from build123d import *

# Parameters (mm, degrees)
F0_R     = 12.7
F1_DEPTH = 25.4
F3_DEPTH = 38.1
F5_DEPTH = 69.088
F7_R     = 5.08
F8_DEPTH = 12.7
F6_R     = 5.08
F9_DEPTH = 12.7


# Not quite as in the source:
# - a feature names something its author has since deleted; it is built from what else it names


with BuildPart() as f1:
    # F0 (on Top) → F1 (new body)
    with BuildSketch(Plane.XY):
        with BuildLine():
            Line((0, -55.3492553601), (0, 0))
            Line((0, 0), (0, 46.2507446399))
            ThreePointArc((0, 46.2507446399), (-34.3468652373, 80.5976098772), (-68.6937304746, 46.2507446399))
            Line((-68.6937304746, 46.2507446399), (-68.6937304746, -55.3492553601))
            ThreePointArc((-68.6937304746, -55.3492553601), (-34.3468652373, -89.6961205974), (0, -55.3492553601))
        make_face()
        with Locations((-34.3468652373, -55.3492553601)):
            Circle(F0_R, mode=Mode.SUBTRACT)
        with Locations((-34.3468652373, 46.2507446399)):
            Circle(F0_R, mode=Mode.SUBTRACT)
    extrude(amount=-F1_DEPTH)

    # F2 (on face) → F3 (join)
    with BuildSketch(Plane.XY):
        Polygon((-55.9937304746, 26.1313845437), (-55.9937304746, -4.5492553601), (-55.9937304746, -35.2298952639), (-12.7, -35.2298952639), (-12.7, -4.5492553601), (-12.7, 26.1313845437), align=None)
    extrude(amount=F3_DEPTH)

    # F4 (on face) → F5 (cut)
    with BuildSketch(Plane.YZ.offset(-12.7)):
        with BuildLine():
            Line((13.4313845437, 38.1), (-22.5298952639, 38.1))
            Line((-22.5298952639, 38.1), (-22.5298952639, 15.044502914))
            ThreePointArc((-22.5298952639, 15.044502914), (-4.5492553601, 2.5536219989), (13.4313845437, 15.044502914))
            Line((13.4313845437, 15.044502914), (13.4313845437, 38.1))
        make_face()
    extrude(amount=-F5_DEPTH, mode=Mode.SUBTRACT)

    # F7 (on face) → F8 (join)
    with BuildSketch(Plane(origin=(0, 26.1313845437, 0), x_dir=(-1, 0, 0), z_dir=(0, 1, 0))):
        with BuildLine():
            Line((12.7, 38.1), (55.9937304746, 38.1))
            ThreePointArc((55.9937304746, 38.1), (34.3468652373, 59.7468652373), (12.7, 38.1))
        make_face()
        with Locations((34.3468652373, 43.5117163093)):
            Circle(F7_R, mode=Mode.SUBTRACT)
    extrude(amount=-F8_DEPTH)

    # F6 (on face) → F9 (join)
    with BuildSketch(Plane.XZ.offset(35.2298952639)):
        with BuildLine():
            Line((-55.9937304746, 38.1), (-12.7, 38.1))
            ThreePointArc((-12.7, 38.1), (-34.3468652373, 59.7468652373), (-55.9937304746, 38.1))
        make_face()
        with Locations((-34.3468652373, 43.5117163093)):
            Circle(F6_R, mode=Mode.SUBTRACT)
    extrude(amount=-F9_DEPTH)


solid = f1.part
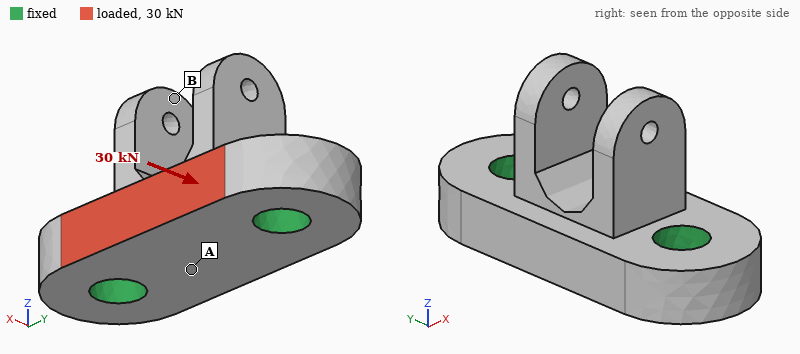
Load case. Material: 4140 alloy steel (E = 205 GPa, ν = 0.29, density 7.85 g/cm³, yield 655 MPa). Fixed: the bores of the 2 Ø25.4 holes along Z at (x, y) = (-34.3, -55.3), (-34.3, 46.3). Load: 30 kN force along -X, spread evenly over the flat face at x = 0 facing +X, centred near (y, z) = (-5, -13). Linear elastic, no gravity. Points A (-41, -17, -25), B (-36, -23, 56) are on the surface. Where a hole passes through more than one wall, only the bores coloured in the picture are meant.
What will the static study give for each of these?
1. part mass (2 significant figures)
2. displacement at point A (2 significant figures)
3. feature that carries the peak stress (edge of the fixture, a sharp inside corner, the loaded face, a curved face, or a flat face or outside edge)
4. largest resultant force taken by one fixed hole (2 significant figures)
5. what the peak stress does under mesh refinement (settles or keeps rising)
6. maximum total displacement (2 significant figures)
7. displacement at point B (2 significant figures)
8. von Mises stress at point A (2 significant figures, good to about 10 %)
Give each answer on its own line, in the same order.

2.5 kg
2.6 µm
edge of the fixture
15 kN
keeps rising
4.5 µm
2.7 µm
7.0 MPa
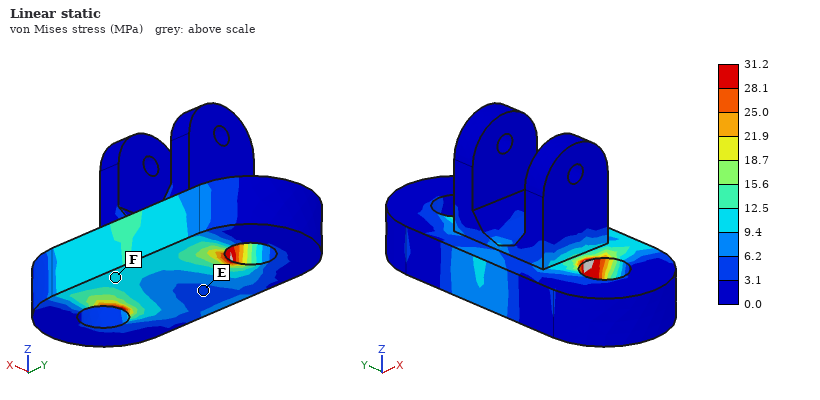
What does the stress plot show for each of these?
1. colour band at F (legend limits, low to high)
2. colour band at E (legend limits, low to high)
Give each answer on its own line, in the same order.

9.4 to 12.5 MPa
3.1 to 6.2 MPa
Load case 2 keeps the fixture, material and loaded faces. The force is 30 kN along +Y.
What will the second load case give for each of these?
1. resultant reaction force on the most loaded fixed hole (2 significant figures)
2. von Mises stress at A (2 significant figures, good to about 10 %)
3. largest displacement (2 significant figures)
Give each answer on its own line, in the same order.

17 kN
3.9 MPa
4.1 µm
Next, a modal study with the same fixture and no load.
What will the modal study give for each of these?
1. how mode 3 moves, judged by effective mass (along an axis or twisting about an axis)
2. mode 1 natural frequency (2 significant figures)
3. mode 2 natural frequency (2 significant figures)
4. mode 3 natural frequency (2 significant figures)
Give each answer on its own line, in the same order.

along X
3900 Hz
4100 Hz
5700 Hz
